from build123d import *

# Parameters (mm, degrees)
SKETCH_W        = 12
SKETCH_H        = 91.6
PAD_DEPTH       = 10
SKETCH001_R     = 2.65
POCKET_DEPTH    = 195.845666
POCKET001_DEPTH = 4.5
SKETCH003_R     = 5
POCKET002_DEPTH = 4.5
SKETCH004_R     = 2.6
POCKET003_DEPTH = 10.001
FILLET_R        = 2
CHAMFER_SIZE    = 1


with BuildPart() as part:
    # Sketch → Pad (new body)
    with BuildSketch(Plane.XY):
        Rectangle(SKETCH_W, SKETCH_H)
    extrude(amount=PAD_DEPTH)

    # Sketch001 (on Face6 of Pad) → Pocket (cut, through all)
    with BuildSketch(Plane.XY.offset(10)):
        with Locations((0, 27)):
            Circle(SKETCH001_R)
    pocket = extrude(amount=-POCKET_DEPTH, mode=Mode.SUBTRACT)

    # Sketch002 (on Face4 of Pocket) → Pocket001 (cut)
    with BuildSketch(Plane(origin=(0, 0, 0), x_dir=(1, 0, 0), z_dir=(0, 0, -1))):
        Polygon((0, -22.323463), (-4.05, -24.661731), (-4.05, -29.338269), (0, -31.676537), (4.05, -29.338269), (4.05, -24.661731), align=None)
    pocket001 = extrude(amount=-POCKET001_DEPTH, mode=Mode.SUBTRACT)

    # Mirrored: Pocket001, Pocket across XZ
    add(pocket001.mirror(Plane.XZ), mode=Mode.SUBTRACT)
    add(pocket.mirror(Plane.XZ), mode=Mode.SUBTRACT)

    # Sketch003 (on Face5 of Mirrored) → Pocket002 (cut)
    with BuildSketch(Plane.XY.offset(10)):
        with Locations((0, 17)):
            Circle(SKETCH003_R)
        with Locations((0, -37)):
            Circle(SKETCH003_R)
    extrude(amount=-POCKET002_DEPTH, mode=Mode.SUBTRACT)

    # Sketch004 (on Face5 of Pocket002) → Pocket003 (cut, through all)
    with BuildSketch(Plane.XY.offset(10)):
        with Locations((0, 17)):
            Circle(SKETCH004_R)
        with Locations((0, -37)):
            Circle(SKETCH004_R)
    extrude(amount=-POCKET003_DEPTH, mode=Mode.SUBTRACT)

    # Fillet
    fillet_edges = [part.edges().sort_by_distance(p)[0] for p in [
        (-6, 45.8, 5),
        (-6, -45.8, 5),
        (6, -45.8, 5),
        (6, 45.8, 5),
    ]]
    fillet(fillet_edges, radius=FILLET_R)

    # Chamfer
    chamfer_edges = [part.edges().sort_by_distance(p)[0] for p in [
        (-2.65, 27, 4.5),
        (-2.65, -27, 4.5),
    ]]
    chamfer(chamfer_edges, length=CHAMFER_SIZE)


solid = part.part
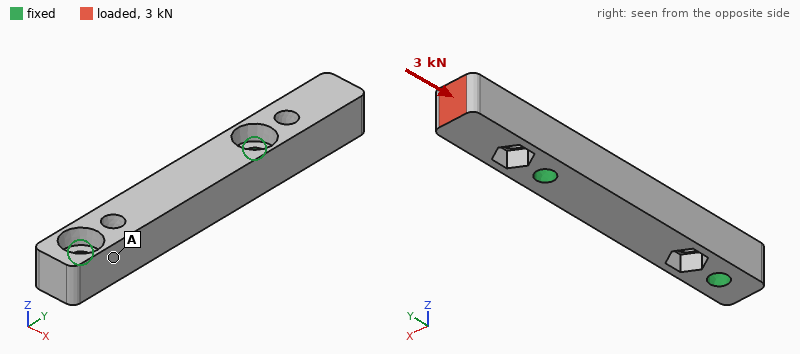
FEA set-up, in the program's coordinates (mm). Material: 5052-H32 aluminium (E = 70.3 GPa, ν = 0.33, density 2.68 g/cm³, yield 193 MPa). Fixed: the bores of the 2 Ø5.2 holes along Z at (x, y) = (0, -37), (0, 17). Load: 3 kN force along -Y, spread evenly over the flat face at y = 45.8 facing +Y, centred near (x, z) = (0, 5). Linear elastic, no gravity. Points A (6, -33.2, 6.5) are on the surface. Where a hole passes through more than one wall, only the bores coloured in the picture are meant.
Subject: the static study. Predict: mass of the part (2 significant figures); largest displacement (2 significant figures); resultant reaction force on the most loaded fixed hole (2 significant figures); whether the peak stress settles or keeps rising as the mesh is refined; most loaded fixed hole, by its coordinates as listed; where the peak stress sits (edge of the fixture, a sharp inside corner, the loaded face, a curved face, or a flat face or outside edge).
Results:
25 g
29 µm
2.8 kN
keeps rising
(0, 17)
a sharp inside corner
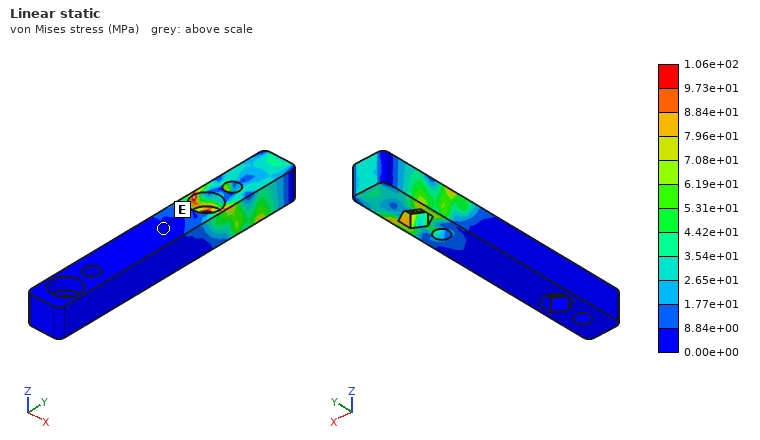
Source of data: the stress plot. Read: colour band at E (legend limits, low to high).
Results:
0.00e+00 to 8.84e+00 MPa
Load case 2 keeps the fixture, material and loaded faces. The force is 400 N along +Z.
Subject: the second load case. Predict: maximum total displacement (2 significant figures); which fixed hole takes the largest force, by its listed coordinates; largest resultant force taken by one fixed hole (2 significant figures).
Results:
0.13 mm
(0, 17)
470 N
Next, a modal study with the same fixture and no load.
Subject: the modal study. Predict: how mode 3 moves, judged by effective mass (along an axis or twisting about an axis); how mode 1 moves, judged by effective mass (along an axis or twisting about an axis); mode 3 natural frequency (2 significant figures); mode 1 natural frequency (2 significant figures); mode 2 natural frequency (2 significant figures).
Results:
along Z
along Z
13 kHz
5800 Hz
7500 Hz
